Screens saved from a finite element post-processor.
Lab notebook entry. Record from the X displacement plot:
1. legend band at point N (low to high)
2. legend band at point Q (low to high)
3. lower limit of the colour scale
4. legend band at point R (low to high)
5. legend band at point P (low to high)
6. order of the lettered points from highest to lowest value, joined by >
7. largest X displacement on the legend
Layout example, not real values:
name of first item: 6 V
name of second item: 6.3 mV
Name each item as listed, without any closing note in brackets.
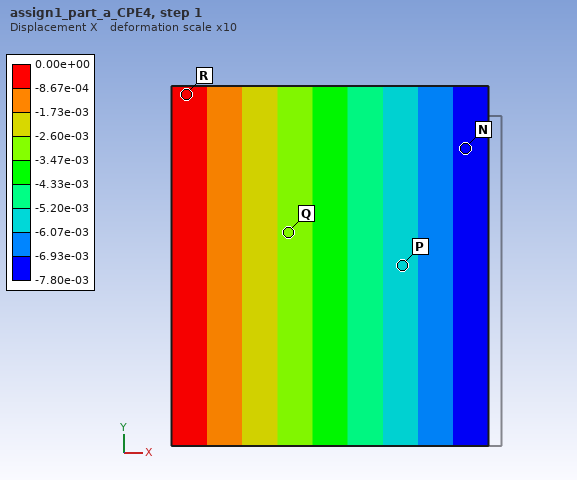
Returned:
legend band at point N: -7.80e-03 to -6.93e-03
legend band at point Q: -3.47e-03 to -2.60e-03
lower limit of the colour scale: -7.80e-03
legend band at point R: -8.67e-04 to 0.00e+00
legend band at point P: -6.07e-03 to -5.20e-03
order of the lettered points from highest to lowest value, joined by >: R > Q > P > N
largest X displacement on the legend: 0.00e+00
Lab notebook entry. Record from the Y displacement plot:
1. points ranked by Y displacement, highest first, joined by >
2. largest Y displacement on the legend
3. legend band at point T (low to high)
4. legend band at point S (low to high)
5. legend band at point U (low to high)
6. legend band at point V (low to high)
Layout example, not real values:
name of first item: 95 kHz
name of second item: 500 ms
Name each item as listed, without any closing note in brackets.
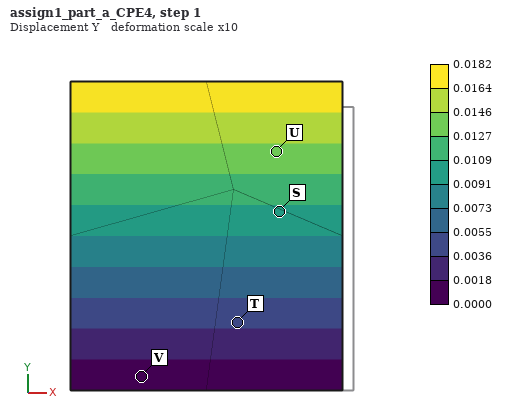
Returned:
points ranked by Y displacement, highest first, joined by >: U > S > T > V
largest Y displacement on the legend: 0.0182
legend band at point T: 0.0036 to 0.0055
legend band at point S: 0.0091 to 0.0109
legend band at point U: 0.0127 to 0.0146
legend band at point V: 0.0000 to 0.0018
